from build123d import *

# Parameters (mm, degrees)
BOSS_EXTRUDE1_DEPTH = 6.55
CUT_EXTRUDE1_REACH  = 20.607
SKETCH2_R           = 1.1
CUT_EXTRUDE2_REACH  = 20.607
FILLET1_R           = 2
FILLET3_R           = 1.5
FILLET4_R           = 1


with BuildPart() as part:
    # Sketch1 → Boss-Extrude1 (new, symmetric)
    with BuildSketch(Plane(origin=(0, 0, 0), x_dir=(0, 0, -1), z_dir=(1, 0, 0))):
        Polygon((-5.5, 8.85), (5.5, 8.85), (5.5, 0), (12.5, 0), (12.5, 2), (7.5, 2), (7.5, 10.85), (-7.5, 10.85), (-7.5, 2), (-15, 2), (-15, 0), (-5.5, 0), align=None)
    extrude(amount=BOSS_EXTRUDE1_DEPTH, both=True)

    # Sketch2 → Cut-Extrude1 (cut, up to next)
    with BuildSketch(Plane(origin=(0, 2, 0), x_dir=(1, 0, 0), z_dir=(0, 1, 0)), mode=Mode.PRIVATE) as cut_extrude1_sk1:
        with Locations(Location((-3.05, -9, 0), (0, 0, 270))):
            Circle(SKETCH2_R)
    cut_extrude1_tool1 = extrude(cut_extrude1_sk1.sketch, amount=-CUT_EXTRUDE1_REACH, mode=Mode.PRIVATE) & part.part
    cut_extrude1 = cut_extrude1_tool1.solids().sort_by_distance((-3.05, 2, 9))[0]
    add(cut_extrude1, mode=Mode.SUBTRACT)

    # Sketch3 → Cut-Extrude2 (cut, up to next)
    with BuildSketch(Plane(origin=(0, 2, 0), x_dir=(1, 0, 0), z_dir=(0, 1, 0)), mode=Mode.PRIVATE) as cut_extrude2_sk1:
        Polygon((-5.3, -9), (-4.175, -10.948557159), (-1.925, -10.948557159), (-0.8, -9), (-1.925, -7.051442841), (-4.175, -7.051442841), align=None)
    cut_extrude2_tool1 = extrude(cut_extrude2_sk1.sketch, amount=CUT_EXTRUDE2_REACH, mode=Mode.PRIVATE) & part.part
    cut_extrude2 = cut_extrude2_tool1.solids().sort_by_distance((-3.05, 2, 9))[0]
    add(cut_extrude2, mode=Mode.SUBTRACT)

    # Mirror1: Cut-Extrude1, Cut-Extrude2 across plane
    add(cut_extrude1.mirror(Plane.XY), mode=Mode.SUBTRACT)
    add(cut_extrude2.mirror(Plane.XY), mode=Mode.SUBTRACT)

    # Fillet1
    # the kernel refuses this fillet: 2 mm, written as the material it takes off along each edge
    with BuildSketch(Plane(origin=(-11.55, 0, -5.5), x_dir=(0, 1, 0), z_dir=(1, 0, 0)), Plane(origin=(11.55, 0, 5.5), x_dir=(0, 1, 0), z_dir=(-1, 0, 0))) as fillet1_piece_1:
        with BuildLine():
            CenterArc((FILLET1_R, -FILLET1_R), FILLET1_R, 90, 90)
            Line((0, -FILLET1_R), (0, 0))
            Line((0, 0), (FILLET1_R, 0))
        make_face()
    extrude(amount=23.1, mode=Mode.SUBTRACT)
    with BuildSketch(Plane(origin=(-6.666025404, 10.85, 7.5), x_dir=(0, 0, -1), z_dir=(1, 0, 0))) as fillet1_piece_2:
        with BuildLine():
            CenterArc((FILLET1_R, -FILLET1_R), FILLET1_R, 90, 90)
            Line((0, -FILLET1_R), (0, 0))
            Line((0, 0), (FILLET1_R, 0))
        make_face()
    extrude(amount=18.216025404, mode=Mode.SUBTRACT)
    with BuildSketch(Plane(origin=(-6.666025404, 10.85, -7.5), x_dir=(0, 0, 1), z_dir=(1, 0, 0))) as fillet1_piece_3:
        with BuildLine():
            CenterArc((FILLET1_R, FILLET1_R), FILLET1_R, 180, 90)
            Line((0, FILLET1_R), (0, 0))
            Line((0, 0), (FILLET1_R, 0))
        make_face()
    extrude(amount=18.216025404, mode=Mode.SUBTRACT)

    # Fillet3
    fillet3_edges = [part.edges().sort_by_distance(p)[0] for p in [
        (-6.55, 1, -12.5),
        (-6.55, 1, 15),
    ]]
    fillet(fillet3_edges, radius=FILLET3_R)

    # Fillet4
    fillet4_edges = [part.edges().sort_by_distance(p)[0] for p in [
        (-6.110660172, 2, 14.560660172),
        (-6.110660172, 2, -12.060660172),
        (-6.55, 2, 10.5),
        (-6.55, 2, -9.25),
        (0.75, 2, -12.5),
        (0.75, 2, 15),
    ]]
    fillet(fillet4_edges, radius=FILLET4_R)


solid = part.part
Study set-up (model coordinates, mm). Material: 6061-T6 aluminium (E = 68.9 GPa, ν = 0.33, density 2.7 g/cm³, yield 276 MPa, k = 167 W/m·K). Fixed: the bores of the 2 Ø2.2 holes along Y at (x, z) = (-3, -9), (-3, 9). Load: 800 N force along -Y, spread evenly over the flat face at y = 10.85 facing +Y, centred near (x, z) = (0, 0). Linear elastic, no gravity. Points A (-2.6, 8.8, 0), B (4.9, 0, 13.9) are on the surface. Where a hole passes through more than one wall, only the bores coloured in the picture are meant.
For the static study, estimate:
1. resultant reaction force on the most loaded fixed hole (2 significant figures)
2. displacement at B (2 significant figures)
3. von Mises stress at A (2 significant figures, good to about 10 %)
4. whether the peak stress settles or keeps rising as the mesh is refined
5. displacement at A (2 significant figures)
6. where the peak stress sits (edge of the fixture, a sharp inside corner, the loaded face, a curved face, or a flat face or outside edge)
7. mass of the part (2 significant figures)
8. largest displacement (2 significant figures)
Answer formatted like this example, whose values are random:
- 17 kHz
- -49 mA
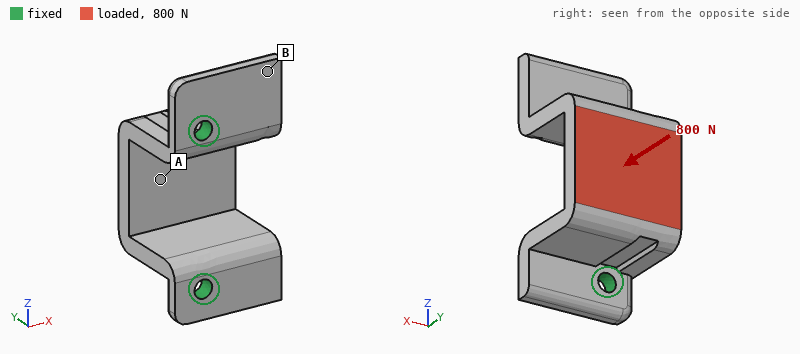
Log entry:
- 430 N
- 23 µm
- 67 MPa
- keeps rising
- 37 µm
- edge of the fixture
- 3.0 g
- 70 µm
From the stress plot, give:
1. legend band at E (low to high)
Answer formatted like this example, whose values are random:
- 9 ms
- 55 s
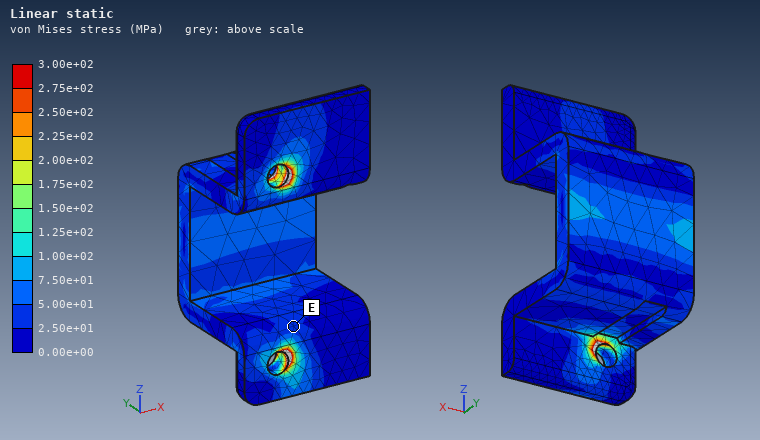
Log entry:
- 2.50e+01 to 5.00e+01 MPa
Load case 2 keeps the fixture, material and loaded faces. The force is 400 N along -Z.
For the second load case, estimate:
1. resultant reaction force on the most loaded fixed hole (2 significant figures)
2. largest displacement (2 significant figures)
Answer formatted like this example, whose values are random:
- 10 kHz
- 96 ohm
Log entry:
- 270 N
- 47 µm
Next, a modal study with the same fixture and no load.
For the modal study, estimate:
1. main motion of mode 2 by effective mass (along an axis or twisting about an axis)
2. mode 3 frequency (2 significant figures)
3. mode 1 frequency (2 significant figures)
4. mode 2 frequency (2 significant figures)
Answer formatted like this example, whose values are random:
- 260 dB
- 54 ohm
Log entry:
- along Z
- 16 kHz
- 9600 Hz
- 13 kHz
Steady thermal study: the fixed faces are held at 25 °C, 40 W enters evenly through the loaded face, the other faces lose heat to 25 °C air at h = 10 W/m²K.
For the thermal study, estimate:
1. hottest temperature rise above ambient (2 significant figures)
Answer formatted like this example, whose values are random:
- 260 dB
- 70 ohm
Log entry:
- 74 K
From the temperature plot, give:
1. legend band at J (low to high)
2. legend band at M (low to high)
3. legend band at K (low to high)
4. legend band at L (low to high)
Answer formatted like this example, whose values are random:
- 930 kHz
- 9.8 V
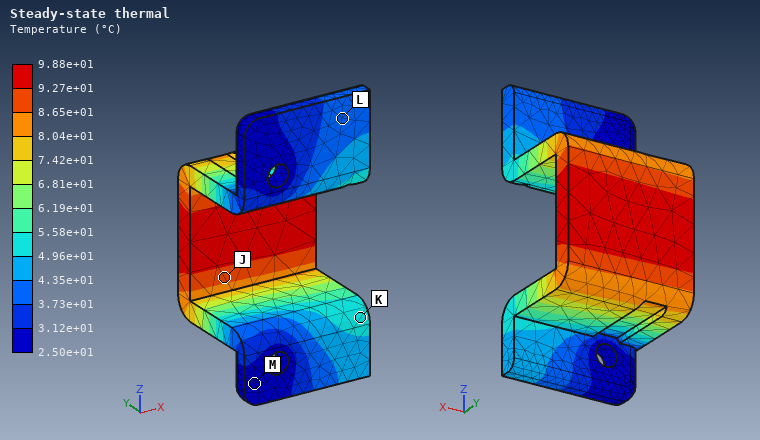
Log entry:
- 8.65e+01 to 9.27e+01 °C
- 2.50e+01 to 3.12e+01 °C
- 4.96e+01 to 5.58e+01 °C
- 3.73e+01 to 4.35e+01 °C
